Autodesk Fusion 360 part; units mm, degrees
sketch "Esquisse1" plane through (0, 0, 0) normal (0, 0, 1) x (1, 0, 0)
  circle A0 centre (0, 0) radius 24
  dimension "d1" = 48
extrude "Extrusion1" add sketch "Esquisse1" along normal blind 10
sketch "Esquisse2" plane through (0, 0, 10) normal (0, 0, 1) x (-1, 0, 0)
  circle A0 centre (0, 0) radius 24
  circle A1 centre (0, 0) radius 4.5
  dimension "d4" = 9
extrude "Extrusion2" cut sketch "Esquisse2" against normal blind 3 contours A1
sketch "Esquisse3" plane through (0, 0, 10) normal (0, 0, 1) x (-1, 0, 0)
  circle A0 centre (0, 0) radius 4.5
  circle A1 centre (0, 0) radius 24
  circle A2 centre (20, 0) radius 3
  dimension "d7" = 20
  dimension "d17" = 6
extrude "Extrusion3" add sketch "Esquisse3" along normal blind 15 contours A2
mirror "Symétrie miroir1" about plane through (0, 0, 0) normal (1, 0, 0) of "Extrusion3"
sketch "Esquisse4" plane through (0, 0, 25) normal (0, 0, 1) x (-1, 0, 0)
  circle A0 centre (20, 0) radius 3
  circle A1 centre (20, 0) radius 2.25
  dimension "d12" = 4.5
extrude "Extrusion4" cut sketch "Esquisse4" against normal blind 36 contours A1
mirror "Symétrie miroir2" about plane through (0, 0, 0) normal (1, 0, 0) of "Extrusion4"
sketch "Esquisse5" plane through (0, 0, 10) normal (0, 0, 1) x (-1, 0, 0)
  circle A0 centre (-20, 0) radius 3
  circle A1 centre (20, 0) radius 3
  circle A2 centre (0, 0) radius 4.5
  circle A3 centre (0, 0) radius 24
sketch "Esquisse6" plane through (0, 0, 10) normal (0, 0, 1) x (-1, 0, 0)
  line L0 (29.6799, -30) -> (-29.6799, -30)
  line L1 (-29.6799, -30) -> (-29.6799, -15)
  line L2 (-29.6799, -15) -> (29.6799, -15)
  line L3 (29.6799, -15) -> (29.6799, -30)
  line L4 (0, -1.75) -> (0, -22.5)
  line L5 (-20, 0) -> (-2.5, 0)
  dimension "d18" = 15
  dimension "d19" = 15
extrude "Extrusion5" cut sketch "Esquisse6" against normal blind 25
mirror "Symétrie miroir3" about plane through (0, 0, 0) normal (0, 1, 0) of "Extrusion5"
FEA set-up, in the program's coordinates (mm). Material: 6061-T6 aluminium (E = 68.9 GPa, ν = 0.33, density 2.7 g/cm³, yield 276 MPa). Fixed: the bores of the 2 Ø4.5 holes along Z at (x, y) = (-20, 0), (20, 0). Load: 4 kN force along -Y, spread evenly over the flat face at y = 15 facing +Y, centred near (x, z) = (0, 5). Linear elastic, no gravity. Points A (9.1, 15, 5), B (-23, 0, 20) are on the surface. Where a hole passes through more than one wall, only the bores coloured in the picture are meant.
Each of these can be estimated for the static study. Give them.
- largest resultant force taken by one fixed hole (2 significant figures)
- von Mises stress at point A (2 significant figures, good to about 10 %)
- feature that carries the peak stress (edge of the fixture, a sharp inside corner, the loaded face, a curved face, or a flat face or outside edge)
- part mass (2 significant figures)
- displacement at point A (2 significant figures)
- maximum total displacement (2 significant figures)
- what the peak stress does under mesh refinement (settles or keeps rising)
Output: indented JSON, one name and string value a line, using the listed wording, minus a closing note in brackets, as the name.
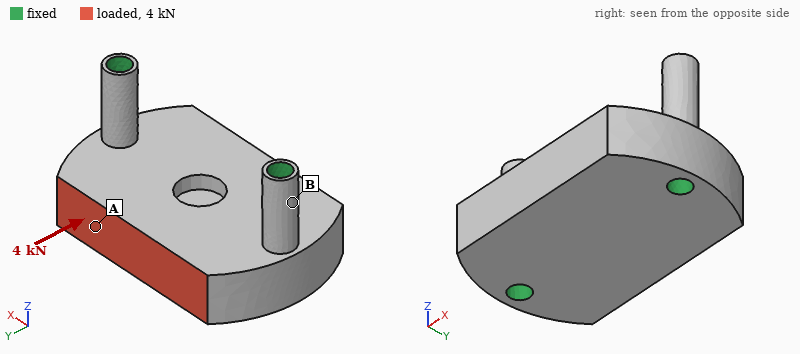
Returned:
{
  "largest resultant force taken by one fixed hole": "2.0 kN",
  "von Mises stress at point A": "12 MPa",
  "feature that carries the peak stress": "edge of the fixture",
  "part mass": "36 g",
  "displacement at point A": "5.4 µm",
  "maximum total displacement": "6.5 µm",
  "what the peak stress does under mesh refinement": "keeps rising"
}
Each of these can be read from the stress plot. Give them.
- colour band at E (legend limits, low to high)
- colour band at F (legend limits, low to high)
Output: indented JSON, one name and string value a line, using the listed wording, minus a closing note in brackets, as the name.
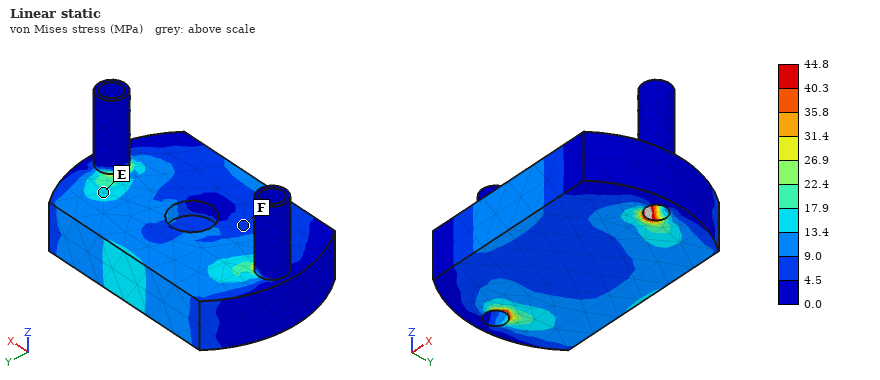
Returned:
{
  "colour band at E": "13.4 to 17.9 MPa",
  "colour band at F": "4.5 to 9.0 MPa"
}
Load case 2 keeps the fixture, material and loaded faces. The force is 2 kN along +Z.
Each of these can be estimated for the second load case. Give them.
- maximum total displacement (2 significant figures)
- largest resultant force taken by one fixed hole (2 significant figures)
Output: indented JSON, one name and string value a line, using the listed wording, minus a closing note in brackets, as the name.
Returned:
{
  "maximum total displacement": "29 µm",
  "largest resultant force taken by one fixed hole": "1.0 kN"
}
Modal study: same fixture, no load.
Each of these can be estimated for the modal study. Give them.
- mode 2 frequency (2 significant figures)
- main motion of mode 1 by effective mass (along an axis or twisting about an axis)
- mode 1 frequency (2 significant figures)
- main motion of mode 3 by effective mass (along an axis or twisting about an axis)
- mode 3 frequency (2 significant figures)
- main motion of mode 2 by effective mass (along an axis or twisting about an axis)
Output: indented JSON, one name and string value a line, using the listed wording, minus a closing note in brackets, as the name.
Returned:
{
  "mode 2 frequency": "19 kHz",
  "main motion of mode 1 by effective mass": "twisting about X",
  "mode 1 frequency": "18 kHz",
  "main motion of mode 3 by effective mass": "along Y",
  "mode 3 frequency": "28 kHz",
  "main motion of mode 2 by effective mass": "along Z"
}
